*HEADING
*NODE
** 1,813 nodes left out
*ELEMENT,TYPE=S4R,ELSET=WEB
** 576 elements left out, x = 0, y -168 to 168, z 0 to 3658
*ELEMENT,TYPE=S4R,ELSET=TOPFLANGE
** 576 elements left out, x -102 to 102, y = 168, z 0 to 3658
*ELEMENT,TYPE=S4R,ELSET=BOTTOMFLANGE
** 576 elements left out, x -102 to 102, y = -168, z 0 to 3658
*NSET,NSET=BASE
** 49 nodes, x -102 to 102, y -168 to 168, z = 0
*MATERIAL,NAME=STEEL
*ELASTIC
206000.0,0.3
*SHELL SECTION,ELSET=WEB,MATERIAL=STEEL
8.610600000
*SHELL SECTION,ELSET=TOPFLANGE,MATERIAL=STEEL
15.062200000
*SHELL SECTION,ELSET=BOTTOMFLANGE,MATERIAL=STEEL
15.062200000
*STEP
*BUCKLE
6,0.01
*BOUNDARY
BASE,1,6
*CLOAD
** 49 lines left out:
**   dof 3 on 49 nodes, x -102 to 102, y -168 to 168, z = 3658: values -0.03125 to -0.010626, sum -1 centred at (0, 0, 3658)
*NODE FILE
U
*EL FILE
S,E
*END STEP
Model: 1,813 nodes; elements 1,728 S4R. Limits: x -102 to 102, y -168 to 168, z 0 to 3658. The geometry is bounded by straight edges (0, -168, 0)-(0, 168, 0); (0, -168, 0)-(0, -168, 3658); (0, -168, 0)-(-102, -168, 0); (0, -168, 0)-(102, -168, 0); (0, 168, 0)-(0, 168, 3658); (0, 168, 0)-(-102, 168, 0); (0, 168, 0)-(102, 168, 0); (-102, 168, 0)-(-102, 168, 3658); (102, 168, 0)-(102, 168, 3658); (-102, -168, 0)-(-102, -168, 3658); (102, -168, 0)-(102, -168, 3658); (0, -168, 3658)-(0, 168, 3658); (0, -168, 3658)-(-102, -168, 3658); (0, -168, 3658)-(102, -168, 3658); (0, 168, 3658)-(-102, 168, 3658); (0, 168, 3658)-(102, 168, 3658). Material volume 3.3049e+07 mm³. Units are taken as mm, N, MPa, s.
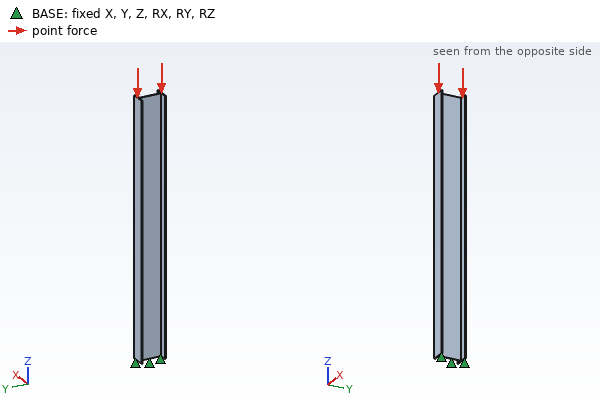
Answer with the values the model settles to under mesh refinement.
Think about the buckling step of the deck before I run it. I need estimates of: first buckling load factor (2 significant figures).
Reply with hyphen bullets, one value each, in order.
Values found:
- 8.0e+05
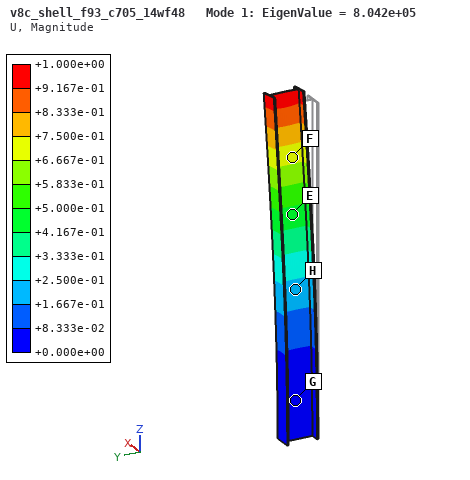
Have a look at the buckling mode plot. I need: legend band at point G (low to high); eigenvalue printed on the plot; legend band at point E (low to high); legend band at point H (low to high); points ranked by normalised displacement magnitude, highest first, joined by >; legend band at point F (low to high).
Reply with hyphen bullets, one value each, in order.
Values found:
- +0.000e+00 to +8.333e-02
- 8.042e+05
- +4.167e-01 to +5.000e-01
- +1.667e-01 to +2.500e-01
- F > E > H > G
- +6.667e-01 to +7.500e-01
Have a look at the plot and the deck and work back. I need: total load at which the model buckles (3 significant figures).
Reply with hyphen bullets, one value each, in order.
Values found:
- 8.04e+05 N
